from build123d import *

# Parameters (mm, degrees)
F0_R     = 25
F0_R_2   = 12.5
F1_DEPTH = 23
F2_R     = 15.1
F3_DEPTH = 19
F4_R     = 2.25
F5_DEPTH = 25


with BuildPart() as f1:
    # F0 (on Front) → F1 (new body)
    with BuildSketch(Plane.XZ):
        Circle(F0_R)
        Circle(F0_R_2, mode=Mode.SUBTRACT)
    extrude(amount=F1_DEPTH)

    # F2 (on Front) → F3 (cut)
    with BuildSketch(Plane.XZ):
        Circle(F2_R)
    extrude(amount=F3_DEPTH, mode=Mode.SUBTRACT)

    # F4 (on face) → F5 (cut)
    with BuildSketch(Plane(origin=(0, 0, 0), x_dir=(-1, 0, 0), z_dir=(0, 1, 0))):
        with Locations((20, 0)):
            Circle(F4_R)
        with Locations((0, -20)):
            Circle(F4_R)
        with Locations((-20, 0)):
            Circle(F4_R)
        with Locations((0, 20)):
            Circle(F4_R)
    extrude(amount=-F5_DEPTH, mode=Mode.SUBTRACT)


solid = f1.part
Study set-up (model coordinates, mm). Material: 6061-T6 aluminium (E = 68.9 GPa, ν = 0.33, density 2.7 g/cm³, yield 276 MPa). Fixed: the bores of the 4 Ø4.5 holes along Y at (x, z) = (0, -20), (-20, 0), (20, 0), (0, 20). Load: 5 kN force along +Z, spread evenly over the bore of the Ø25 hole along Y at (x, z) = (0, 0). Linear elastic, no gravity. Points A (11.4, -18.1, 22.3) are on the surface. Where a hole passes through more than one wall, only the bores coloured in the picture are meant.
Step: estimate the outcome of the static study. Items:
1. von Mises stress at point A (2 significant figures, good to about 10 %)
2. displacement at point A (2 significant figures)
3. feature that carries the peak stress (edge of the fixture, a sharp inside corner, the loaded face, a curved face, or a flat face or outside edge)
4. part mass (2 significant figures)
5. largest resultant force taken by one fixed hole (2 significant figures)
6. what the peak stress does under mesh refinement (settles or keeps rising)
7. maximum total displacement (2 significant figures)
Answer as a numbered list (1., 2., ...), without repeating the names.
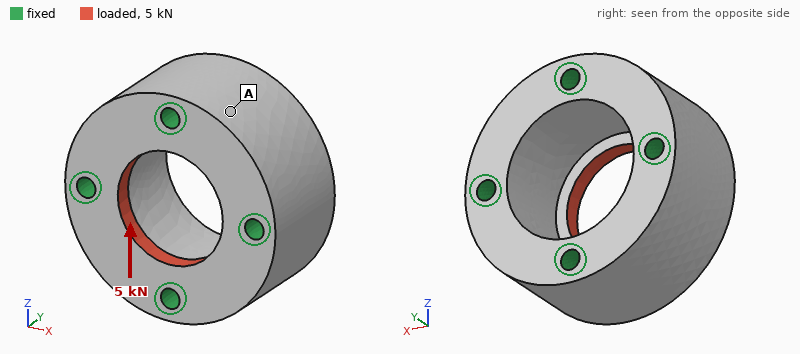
1. 6.0 MPa
2. 1.6 µm
3. edge of the fixture
4. 76 g
5. 1.3 kN
6. keeps rising
7. 4.3 µm
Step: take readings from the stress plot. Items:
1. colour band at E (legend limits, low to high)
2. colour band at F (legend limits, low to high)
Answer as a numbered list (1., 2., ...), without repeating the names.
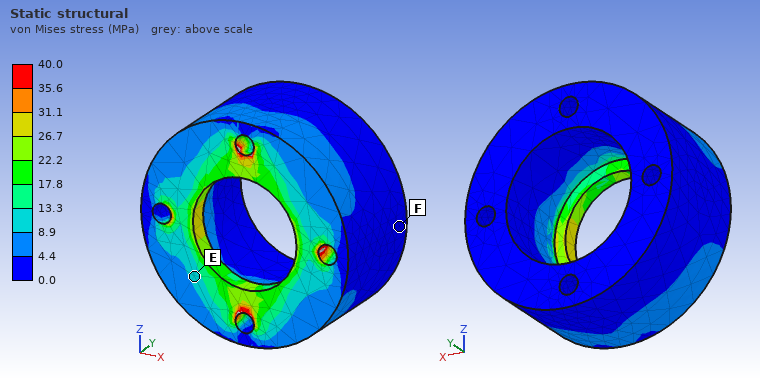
1. 8.9 to 13.3 MPa
2. 0.0 to 4.4 MPa
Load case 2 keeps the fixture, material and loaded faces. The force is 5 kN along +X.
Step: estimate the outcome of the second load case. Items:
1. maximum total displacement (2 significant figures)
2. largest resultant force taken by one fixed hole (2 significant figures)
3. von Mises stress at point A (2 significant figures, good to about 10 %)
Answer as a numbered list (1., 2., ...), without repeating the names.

1. 4.3 µm
2. 1.4 kN
3. 5.2 MPa
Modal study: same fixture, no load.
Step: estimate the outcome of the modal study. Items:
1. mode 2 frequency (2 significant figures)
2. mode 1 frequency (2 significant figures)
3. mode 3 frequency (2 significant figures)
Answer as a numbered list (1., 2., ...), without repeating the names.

1. 43 kHz
2. 42 kHz
3. 43 kHz
